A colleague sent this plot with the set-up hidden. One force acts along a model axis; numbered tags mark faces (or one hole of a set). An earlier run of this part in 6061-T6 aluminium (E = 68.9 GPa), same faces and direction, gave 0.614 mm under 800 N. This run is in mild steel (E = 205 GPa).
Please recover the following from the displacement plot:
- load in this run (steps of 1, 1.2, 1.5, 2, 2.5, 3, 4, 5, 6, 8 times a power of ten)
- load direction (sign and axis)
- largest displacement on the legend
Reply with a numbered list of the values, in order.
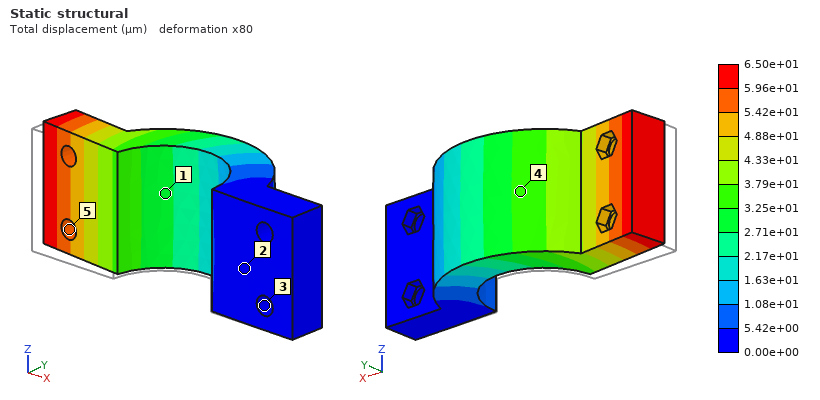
1. 250 N
2. +Y
3. 6.50e+01 µm
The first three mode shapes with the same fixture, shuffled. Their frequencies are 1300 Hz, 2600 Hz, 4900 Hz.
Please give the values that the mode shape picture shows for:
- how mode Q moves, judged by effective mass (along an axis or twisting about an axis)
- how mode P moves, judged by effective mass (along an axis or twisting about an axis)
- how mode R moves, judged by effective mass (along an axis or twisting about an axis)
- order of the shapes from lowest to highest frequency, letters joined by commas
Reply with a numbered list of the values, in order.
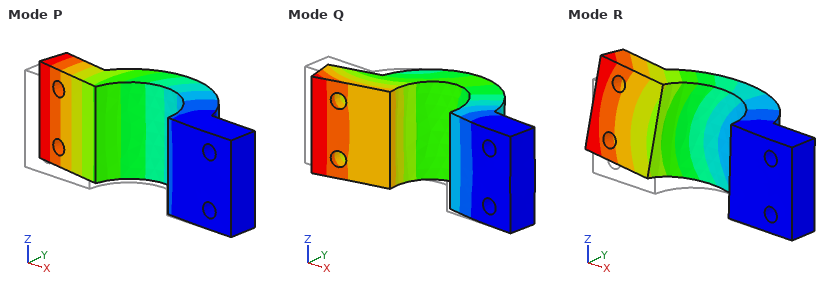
1. along X
2. along Y
3. along Z
4. P, R, Q
